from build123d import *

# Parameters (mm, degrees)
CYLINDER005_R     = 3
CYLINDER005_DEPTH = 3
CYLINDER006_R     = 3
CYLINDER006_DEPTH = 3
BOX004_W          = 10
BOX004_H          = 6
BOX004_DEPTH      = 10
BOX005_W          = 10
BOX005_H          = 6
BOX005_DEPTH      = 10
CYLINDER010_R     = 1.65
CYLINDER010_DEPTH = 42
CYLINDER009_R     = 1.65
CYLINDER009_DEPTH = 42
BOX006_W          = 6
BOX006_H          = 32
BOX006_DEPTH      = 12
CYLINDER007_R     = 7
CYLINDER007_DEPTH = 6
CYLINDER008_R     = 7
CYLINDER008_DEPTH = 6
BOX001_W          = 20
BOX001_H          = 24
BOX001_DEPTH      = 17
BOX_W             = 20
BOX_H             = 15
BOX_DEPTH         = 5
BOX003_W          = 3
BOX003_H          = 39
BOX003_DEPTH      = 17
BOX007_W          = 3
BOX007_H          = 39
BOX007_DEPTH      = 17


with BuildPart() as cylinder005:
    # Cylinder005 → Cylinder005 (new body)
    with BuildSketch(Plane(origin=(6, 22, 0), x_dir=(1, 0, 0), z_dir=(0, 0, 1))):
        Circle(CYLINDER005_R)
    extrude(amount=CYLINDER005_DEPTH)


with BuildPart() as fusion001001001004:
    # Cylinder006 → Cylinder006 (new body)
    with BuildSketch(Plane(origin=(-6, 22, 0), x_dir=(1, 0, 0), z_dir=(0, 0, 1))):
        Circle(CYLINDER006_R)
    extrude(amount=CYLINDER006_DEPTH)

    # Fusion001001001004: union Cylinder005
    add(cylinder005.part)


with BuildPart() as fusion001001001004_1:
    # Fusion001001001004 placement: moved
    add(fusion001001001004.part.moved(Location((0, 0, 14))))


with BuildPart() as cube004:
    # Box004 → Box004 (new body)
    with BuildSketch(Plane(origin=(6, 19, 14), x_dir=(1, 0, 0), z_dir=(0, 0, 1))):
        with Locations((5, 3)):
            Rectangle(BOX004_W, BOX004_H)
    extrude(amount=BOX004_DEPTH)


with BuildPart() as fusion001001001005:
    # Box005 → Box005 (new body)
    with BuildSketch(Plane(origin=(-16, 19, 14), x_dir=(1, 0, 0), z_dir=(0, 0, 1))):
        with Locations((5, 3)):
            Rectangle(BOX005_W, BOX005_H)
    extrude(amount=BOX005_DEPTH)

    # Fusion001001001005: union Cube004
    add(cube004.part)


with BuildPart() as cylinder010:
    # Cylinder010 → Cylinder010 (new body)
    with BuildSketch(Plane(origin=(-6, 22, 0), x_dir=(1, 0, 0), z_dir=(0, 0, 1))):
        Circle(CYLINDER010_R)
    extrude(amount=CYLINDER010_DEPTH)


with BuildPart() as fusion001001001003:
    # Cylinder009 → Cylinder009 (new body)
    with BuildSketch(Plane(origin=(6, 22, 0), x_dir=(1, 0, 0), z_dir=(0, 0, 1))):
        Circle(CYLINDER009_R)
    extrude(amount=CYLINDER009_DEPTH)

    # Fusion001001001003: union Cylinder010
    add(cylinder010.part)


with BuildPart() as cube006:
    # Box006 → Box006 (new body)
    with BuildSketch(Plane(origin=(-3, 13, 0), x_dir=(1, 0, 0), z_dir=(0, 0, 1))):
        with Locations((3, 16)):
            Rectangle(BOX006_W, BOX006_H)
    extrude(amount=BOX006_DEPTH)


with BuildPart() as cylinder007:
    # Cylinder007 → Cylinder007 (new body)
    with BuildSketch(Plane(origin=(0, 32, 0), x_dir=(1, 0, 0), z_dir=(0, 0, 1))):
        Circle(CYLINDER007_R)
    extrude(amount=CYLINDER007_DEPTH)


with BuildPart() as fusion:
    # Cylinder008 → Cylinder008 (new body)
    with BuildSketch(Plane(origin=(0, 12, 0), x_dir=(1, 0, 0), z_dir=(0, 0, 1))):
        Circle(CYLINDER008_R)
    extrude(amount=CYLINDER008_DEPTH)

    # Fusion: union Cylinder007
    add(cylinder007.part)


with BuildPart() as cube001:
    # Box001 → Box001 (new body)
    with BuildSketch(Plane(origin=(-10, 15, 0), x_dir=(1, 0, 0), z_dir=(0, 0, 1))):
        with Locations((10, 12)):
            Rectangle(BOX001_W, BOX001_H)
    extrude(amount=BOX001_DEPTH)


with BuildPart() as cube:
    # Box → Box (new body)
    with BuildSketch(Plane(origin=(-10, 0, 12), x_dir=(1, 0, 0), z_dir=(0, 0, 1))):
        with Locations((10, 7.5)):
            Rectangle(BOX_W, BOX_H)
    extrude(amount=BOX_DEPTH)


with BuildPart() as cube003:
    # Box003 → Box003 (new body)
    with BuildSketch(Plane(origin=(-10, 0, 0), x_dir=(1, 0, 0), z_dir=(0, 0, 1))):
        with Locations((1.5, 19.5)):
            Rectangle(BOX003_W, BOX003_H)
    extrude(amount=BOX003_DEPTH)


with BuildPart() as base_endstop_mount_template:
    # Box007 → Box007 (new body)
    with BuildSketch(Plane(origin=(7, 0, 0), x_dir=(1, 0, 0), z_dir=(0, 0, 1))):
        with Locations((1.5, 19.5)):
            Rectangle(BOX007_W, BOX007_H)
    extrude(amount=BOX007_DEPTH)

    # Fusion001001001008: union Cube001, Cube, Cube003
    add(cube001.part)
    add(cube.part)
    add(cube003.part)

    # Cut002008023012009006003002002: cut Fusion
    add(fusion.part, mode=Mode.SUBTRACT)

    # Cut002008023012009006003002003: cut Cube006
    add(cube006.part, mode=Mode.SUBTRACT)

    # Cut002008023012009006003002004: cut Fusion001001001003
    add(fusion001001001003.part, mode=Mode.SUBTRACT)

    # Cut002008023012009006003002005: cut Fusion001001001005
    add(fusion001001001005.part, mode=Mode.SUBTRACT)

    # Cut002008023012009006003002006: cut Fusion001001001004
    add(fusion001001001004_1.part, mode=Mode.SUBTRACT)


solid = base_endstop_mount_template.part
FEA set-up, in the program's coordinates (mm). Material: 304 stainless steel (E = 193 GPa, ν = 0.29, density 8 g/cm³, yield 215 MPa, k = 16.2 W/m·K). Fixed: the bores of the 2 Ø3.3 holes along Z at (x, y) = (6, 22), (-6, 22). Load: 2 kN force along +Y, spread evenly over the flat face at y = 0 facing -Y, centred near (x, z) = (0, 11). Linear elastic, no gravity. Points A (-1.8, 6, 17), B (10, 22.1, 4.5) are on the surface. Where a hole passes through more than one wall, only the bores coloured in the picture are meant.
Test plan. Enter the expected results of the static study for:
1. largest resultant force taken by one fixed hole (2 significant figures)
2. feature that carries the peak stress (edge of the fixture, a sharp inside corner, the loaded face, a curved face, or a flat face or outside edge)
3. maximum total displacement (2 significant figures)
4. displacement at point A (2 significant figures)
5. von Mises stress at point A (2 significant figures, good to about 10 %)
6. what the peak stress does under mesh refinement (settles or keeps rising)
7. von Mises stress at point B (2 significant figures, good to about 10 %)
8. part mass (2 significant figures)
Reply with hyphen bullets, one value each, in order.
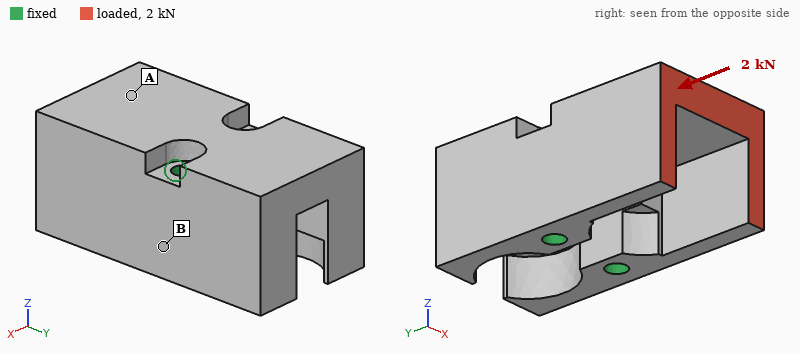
- 1.0 kN
- edge of the fixture
- 2.1 µm
- 1.7 µm
- 12 MPa
- keeps rising
- 4.9 MPa
- 64 g
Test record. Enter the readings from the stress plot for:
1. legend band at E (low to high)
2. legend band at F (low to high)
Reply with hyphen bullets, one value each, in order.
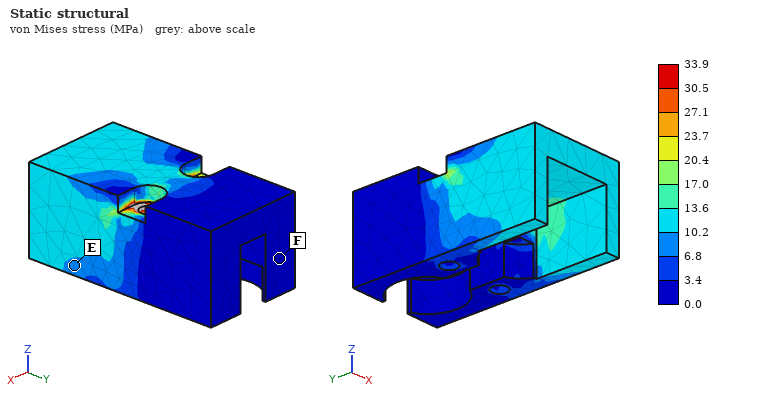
- 6.8 to 10.2 MPa
- 0.0 to 3.4 MPa
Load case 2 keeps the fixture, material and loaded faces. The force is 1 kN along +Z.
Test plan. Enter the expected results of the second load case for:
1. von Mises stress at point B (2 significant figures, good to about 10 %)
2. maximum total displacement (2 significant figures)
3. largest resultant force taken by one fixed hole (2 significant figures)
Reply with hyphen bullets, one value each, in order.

- 12 MPa
- 11 µm
- 500 N
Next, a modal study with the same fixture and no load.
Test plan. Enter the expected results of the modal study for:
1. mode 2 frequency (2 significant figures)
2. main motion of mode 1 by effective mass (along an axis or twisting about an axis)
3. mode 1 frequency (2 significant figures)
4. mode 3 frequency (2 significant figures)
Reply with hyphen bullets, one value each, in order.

- 17 kHz
- along X
- 14 kHz
- 19 kHz
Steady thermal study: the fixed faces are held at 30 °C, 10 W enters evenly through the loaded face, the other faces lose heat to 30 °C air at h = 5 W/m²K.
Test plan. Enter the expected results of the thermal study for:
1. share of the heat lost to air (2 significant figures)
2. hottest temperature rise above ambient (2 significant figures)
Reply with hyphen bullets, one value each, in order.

- 3.9 %
- 74 K
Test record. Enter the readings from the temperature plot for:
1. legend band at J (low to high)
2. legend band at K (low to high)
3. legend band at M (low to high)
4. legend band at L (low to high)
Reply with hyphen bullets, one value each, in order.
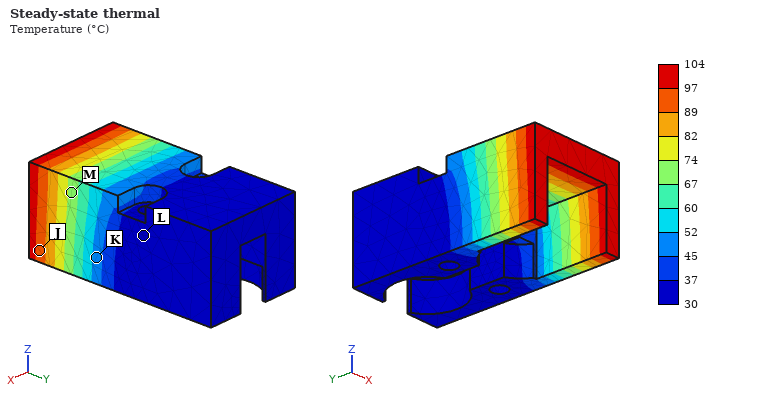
- 89 to 97 °C
- 45 to 52 °C
- 67 to 74 °C
- 30 to 37 °C
